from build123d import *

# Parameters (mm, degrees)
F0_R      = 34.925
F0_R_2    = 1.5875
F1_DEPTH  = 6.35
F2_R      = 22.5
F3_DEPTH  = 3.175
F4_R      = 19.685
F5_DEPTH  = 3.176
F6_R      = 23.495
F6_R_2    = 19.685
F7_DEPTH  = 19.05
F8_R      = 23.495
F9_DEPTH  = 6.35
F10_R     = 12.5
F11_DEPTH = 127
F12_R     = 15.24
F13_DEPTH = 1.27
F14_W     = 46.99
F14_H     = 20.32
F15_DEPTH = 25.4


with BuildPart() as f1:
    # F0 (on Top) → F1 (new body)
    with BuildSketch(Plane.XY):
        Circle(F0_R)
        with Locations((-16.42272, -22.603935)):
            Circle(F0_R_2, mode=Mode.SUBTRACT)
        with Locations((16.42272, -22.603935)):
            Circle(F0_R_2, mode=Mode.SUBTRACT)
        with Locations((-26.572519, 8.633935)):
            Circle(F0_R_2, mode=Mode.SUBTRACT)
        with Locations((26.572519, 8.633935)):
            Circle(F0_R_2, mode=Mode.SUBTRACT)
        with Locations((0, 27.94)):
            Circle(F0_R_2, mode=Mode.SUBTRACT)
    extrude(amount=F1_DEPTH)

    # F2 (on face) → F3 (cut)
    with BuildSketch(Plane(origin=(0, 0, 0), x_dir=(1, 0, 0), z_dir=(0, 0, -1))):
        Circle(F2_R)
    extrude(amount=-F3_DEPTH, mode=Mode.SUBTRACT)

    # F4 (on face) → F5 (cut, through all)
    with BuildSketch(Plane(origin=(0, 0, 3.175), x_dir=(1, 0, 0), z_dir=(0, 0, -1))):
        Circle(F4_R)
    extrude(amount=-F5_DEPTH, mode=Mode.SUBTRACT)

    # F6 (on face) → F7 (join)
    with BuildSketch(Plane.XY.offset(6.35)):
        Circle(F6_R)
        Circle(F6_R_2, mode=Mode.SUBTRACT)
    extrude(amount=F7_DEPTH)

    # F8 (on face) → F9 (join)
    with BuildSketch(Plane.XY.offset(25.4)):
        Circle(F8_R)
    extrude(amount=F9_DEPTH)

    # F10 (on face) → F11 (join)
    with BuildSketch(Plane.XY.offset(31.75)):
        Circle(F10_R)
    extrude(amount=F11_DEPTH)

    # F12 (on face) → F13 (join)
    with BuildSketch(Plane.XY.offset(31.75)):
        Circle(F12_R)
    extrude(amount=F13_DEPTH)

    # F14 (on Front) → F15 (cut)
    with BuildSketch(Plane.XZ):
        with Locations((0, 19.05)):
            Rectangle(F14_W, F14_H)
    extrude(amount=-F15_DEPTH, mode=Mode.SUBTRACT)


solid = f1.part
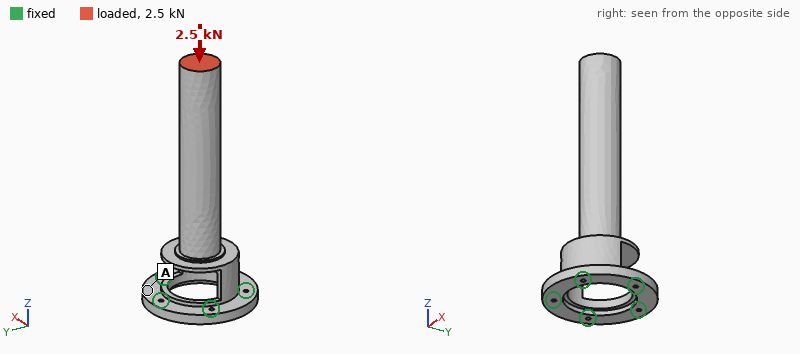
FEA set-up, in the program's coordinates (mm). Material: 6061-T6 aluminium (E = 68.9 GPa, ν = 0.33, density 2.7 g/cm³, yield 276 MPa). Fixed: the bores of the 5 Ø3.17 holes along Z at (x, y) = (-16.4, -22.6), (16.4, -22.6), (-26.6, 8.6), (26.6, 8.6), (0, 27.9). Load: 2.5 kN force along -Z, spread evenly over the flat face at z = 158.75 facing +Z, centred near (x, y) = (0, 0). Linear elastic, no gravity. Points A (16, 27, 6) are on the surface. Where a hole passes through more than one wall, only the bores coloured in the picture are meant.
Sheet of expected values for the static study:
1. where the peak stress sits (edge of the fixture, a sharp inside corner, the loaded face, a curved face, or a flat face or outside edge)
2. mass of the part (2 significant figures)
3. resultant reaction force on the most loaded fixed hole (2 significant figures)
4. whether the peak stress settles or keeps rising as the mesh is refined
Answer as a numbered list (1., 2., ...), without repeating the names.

1. edge of the fixture
2. 250 g
3. 1.0 kN
4. keeps rising
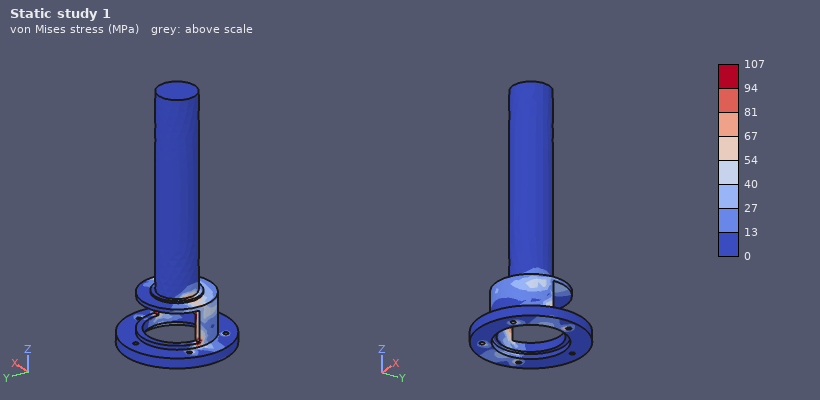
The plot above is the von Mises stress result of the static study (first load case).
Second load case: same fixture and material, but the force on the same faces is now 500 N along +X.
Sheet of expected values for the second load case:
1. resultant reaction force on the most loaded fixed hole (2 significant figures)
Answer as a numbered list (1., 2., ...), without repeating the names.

1. 1.4 kN
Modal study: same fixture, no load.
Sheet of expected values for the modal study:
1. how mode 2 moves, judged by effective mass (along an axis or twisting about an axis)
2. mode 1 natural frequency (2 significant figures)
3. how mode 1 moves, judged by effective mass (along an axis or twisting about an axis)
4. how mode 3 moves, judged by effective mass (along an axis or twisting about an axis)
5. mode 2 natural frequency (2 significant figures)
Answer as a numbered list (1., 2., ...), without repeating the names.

1. along X
2. 370 Hz
3. along Y
4. along X
5. 640 Hz
